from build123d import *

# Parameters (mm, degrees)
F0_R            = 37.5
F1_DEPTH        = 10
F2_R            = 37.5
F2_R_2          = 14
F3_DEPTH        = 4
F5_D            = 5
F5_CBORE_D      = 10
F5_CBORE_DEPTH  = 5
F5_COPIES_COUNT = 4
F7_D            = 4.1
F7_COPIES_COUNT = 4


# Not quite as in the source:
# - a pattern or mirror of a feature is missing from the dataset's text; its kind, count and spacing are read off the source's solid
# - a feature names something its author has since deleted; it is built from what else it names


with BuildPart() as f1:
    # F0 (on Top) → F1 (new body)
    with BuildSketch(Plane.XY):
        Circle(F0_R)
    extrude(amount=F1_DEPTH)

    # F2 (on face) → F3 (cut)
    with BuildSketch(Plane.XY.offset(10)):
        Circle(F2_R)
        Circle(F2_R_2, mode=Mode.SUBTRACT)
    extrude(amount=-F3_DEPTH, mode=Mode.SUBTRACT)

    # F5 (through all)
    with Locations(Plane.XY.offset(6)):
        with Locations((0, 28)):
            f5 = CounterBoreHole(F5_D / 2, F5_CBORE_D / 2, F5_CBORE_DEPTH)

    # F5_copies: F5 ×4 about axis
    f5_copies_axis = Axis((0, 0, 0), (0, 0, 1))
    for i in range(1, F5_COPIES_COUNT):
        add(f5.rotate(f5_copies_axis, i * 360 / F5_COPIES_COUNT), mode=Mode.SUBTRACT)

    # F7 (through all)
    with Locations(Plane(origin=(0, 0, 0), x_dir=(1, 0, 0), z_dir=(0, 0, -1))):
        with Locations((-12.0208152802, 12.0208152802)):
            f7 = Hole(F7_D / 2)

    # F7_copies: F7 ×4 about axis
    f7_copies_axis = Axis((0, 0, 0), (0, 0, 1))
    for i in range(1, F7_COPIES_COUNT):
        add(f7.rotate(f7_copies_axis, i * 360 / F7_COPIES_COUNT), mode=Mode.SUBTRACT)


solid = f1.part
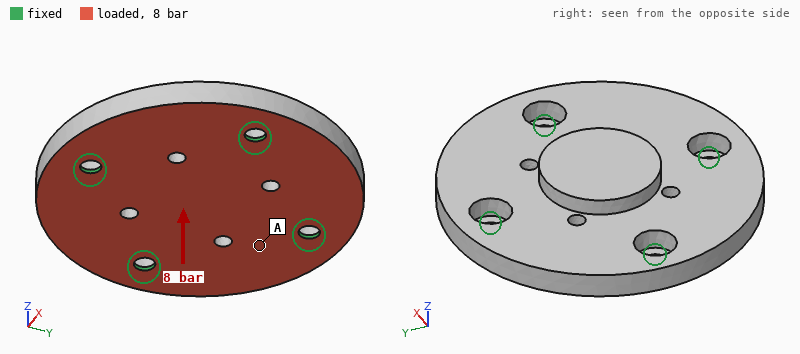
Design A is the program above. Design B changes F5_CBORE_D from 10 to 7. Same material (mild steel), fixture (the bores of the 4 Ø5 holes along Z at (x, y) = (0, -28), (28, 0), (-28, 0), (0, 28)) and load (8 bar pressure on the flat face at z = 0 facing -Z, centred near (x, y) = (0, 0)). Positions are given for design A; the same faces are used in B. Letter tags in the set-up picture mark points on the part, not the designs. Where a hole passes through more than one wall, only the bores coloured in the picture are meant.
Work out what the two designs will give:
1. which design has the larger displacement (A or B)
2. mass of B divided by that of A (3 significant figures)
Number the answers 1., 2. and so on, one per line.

1. A
2. 1.03
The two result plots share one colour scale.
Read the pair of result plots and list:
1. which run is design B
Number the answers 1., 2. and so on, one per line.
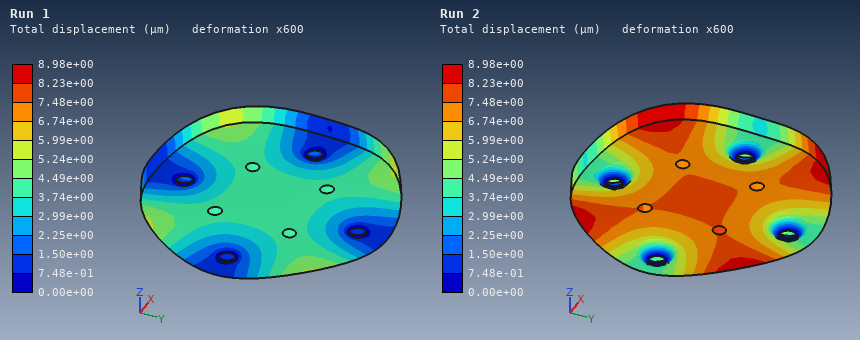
1. Run 1
